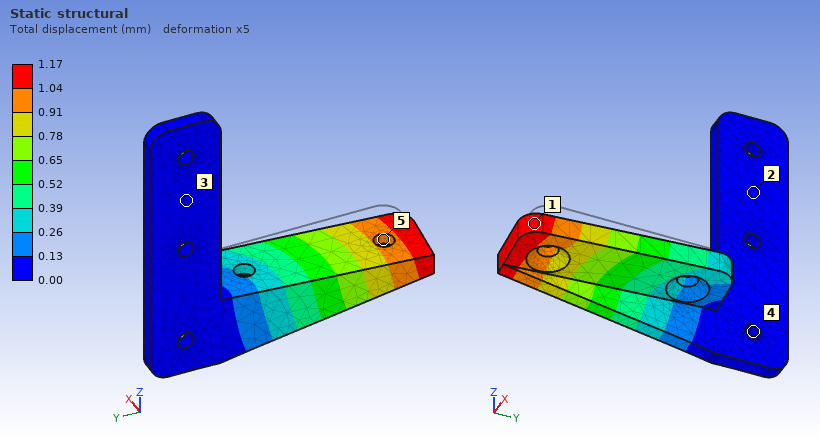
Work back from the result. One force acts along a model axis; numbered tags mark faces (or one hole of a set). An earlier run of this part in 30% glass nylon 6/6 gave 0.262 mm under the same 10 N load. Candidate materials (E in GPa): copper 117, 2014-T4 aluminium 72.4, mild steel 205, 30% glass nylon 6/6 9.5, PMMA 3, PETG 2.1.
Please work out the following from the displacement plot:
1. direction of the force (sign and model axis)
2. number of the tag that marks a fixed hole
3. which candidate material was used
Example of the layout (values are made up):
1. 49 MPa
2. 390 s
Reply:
1. -X
2. 4
3. PETG
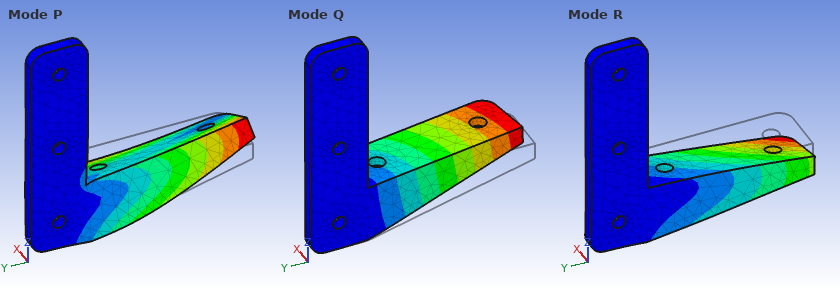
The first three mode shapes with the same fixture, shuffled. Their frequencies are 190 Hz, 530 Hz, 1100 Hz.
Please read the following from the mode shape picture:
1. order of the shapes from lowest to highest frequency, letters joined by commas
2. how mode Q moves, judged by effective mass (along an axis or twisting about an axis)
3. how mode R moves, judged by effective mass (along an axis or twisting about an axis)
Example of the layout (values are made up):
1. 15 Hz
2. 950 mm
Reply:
1. Q, R, P
2. along X
3. along Z
